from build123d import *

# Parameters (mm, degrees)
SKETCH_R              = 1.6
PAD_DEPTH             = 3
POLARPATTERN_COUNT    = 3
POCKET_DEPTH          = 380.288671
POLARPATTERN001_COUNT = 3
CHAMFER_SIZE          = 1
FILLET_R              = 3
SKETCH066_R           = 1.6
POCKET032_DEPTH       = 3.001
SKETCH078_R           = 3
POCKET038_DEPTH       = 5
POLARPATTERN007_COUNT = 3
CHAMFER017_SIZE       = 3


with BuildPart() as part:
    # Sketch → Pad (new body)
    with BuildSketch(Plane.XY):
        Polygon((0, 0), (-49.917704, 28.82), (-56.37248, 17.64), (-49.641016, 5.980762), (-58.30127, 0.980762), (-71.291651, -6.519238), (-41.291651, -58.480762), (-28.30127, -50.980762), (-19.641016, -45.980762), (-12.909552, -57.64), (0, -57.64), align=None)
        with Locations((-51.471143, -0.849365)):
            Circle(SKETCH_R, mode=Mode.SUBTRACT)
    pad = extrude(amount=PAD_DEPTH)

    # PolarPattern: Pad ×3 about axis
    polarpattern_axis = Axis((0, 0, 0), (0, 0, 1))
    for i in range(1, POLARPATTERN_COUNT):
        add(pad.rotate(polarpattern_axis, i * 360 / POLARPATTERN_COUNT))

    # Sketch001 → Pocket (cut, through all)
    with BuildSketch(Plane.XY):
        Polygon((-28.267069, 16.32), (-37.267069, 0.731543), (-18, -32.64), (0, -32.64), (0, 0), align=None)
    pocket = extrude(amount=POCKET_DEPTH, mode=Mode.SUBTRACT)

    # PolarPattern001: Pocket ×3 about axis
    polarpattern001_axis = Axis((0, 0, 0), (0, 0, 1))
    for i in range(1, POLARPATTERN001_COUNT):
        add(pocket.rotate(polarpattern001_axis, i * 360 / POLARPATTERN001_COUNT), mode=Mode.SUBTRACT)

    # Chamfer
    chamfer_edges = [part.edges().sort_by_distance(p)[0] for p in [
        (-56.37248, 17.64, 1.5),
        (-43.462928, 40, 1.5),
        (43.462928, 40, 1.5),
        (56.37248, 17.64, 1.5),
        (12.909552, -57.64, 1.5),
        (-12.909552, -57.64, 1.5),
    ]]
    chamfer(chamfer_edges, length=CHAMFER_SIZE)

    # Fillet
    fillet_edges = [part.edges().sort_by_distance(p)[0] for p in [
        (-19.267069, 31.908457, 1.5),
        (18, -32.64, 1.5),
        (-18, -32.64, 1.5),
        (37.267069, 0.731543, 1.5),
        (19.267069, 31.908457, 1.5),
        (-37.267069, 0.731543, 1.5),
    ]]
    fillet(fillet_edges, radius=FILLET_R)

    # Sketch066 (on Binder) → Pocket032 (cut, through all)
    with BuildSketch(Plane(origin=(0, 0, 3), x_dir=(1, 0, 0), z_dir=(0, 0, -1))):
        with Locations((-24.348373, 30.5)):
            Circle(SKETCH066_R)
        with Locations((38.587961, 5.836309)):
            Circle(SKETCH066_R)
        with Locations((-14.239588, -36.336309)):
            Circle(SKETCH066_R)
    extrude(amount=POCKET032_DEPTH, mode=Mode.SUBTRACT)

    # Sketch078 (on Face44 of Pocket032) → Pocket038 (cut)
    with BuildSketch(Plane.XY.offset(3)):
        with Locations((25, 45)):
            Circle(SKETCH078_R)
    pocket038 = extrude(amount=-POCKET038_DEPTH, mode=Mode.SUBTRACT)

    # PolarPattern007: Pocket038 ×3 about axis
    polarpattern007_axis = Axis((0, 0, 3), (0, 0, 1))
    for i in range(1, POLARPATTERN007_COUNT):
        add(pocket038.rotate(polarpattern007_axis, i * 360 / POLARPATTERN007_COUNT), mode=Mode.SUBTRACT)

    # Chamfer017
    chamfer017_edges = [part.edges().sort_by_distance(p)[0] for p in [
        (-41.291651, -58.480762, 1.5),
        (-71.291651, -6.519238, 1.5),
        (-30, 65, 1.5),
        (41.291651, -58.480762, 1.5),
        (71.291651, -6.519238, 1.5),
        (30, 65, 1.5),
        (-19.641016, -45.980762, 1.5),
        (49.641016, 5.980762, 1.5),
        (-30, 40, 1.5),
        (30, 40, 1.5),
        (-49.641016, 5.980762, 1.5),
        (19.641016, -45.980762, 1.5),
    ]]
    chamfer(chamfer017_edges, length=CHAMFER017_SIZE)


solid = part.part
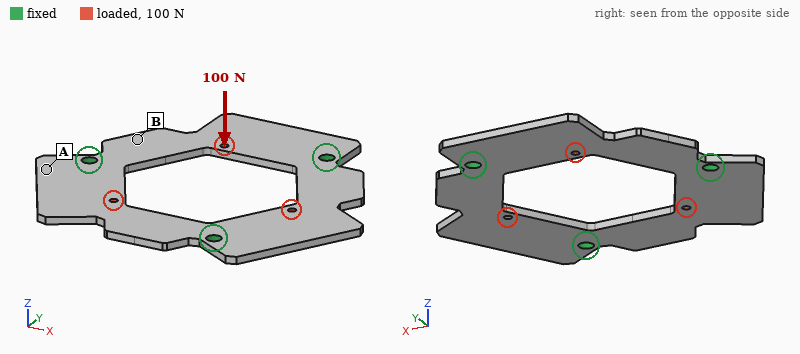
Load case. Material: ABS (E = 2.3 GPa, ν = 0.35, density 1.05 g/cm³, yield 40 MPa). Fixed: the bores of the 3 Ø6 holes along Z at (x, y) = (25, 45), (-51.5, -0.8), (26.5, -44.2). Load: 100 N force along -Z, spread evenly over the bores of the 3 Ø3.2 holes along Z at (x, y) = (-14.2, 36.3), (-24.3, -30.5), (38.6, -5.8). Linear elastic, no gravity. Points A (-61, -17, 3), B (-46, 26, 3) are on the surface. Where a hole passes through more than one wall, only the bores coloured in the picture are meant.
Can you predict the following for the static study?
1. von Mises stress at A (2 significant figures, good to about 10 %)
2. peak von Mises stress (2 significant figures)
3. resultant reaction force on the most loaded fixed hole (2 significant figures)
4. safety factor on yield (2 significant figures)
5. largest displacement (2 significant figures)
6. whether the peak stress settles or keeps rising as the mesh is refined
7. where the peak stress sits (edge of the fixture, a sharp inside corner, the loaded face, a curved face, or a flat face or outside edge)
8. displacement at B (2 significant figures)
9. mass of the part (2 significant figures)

4.2 MPa
28 MPa
33 N
1.4
1.4 mm
settles
the loaded face
0.56 mm
26 g
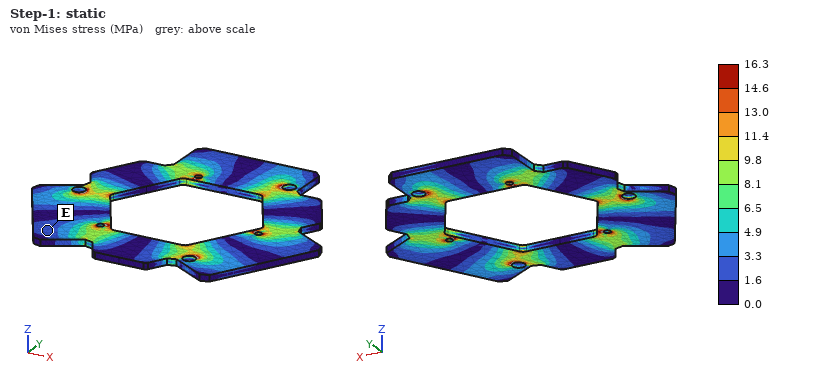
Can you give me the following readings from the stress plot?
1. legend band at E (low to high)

1.6 to 3.3 MPa
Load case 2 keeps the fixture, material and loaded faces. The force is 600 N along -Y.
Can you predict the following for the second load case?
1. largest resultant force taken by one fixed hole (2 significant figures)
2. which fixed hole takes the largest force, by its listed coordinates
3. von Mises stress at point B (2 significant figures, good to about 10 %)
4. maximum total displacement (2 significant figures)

320 N
(-51.5, -0.8)
1.4 MPa
0.14 mm
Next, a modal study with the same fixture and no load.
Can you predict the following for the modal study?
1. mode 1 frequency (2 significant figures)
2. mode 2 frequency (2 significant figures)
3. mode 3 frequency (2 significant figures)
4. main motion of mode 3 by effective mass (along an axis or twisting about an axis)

340 Hz
340 Hz
360 Hz
along Z
